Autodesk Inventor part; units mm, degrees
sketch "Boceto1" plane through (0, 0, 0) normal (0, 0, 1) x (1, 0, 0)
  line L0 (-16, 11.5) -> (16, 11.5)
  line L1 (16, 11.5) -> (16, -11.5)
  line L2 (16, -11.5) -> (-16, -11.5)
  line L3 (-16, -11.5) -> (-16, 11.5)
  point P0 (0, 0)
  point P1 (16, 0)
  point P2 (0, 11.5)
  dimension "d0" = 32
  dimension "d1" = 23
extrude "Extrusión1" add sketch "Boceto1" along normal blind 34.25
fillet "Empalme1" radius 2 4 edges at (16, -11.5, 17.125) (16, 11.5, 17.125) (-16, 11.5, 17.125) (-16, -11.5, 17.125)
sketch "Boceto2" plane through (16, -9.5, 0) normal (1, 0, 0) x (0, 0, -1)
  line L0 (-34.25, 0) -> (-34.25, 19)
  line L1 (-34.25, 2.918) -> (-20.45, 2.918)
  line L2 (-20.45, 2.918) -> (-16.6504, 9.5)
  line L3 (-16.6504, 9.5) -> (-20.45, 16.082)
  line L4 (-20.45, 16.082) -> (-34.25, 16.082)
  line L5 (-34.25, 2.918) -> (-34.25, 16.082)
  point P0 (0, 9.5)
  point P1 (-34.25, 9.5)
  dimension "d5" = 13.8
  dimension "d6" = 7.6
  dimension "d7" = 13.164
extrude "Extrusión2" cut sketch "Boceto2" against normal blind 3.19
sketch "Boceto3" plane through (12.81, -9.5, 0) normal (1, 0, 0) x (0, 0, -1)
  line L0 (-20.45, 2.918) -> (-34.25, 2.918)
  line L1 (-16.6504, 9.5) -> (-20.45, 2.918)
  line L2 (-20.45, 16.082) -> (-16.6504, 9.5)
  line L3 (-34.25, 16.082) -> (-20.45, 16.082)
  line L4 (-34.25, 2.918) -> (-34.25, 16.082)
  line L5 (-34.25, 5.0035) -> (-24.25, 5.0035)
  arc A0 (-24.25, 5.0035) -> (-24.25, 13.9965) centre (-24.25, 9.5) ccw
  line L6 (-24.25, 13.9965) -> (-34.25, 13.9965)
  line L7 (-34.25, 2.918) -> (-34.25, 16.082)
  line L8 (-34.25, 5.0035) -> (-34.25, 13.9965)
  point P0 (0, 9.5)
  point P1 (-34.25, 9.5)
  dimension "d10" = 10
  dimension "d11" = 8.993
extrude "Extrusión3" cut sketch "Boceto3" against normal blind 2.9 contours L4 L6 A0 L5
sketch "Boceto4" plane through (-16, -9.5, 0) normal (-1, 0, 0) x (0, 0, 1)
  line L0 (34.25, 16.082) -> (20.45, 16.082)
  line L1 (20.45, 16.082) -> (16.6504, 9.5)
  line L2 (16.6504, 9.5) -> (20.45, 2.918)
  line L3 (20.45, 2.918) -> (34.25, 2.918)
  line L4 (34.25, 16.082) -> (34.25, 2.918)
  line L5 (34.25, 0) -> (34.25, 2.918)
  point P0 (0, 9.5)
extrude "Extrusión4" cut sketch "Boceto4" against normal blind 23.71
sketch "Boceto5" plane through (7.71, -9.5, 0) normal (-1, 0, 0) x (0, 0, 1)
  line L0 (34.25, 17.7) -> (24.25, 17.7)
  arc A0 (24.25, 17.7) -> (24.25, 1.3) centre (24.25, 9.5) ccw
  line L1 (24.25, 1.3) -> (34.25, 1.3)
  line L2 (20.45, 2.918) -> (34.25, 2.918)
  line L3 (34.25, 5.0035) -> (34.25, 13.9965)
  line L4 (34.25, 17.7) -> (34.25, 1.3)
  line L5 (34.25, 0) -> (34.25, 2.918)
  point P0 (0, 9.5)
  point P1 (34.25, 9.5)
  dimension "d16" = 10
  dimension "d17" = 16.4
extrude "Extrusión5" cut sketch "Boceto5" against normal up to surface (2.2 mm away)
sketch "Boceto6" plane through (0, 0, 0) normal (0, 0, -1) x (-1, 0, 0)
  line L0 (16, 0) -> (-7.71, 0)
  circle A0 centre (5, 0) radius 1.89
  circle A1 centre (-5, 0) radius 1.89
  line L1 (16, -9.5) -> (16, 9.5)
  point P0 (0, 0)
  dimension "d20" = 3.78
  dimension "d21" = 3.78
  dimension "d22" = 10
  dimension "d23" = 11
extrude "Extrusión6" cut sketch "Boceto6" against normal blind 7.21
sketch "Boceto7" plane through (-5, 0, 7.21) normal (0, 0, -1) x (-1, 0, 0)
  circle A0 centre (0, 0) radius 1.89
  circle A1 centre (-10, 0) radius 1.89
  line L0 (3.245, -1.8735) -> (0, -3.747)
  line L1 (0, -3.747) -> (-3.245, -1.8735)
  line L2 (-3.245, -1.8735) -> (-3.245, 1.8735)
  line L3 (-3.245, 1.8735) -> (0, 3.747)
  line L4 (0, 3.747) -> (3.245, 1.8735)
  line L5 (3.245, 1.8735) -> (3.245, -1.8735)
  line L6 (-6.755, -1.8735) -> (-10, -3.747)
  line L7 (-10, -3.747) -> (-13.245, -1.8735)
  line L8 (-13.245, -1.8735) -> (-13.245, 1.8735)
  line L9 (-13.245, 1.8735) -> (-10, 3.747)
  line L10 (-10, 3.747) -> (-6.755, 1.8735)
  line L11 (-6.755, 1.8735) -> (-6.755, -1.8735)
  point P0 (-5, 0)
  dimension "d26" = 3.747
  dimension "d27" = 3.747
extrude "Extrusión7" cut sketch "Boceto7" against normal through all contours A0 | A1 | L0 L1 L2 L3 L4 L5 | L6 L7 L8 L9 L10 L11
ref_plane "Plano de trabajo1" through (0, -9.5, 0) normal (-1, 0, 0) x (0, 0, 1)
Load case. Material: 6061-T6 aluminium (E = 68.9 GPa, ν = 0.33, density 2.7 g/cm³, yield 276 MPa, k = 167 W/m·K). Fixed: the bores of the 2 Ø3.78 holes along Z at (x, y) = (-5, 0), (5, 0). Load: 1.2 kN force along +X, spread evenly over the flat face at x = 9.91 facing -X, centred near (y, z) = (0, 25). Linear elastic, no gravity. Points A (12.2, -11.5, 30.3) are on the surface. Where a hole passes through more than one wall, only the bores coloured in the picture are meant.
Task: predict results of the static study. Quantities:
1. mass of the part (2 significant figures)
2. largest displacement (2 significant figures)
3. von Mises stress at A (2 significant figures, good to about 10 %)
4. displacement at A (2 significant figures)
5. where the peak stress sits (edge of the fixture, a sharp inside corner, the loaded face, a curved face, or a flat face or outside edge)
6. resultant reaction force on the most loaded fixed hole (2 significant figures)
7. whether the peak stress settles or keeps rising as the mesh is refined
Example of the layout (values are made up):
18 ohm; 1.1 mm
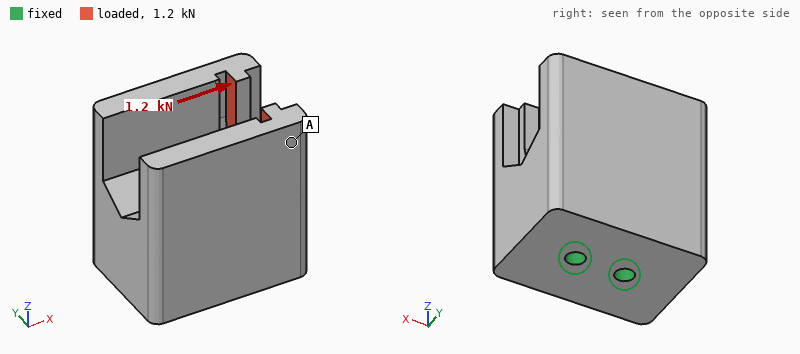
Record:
48 g; 28 µm; 10 MPa; 16 µm; edge of the fixture; 1.6 kN; keeps rising
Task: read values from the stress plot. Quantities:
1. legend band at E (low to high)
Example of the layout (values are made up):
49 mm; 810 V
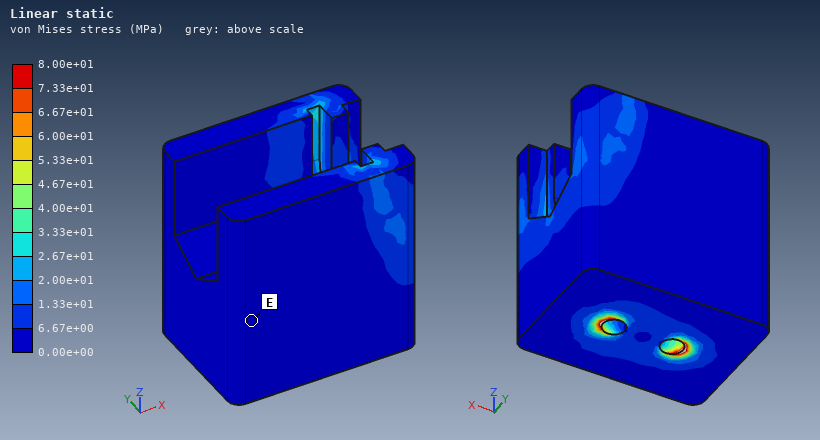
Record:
0.00e+00 to 6.67e+00 MPa
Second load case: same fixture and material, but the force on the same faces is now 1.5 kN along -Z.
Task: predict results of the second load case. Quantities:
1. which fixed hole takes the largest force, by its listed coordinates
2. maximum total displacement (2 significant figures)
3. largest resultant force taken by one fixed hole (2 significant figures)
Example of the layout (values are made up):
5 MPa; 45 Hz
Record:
(5, 0); 14 µm; 1.7 kN
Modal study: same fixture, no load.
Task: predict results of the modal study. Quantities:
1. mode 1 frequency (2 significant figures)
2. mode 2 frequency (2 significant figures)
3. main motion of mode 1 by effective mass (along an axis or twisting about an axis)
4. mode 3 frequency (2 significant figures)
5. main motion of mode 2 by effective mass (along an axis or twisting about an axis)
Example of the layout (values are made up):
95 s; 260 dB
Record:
6500 Hz; 9600 Hz; along Y; 13 kHz; along X
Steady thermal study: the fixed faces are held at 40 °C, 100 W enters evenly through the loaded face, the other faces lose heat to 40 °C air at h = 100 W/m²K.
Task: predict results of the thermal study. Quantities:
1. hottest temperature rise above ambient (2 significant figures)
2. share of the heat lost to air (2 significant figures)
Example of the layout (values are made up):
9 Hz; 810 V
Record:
58 K; 11 %
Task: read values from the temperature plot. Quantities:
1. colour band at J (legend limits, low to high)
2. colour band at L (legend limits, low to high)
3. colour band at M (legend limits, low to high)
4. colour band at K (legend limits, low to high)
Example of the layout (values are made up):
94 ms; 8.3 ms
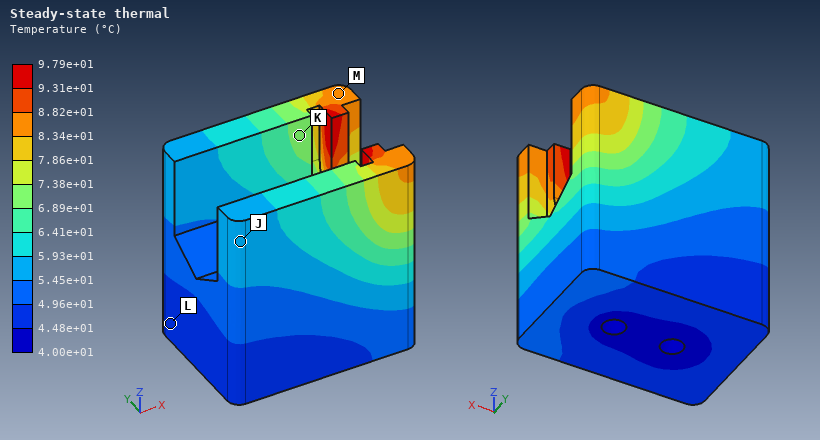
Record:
5.45e+01 to 5.93e+01 °C; 4.48e+01 to 4.96e+01 °C; 8.34e+01 to 8.82e+01 °C; 6.89e+01 to 7.38e+01 °C
